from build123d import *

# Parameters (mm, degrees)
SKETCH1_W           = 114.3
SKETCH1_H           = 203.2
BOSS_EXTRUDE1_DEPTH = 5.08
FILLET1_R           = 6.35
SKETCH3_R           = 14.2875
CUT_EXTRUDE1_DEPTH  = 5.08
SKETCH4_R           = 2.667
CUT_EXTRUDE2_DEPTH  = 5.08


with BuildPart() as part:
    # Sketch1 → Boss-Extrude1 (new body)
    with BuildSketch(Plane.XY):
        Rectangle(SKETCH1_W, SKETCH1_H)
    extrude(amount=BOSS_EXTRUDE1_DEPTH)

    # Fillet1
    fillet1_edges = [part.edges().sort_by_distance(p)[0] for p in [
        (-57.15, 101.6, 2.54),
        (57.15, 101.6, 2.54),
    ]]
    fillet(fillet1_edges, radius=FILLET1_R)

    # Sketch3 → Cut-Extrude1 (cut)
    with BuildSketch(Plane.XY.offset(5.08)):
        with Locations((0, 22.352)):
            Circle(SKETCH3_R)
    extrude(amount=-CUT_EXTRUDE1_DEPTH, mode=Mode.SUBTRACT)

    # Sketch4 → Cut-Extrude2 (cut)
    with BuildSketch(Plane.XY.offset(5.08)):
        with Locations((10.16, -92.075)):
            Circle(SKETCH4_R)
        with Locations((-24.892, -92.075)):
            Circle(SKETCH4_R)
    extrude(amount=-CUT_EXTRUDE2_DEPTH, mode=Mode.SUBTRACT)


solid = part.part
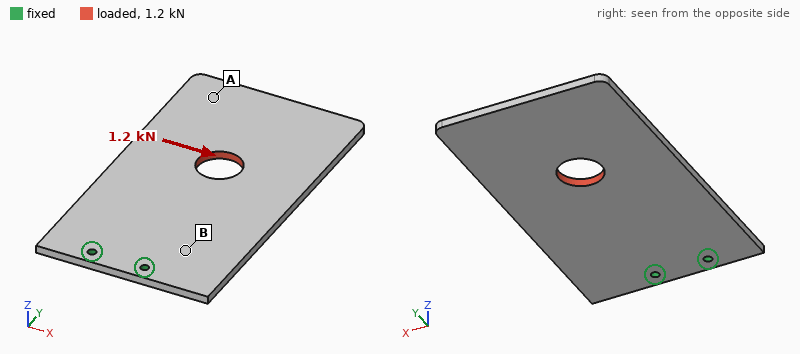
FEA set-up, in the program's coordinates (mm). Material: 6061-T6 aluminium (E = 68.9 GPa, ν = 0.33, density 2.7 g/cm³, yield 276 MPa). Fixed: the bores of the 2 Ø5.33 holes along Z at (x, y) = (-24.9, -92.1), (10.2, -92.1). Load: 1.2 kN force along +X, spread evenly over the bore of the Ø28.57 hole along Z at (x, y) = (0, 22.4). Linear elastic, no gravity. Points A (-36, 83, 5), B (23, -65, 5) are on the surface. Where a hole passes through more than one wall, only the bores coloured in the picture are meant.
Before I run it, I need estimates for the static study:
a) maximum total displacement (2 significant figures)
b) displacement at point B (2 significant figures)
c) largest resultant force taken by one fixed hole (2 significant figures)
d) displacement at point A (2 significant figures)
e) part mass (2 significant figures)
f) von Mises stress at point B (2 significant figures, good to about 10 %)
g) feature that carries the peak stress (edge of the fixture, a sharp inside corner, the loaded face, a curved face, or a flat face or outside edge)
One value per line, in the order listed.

0.16 mm
0.028 mm
3.6 kN
0.14 mm
310 g
10 MPa
edge of the fixture
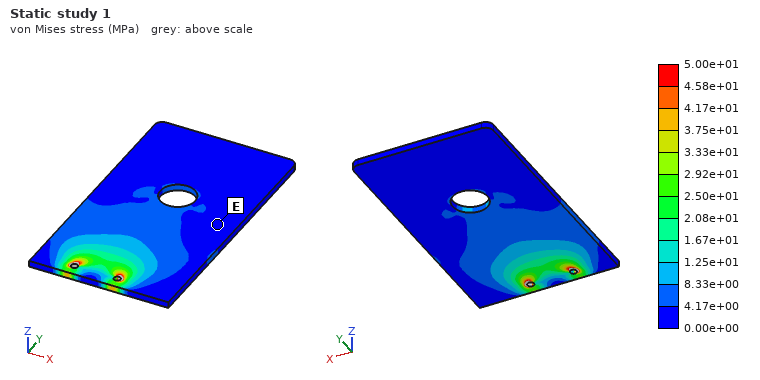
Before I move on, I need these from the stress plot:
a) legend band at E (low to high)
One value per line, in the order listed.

0.00e+00 to 4.17e+00 MPa
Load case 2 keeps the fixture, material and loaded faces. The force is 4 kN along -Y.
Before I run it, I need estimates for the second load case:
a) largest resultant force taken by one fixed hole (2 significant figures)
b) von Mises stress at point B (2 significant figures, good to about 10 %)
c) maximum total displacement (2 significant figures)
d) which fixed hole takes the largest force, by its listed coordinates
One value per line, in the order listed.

2.8 kN
11 MPa
39 µm
(10.2, -92.1)
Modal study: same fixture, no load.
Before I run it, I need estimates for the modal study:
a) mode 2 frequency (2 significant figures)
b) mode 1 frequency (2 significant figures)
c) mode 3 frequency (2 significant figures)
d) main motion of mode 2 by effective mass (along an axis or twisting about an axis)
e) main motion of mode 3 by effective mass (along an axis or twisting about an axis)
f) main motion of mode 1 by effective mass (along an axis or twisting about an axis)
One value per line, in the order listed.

360 Hz
110 Hz
630 Hz
twisting about Y
along Z
along Z
